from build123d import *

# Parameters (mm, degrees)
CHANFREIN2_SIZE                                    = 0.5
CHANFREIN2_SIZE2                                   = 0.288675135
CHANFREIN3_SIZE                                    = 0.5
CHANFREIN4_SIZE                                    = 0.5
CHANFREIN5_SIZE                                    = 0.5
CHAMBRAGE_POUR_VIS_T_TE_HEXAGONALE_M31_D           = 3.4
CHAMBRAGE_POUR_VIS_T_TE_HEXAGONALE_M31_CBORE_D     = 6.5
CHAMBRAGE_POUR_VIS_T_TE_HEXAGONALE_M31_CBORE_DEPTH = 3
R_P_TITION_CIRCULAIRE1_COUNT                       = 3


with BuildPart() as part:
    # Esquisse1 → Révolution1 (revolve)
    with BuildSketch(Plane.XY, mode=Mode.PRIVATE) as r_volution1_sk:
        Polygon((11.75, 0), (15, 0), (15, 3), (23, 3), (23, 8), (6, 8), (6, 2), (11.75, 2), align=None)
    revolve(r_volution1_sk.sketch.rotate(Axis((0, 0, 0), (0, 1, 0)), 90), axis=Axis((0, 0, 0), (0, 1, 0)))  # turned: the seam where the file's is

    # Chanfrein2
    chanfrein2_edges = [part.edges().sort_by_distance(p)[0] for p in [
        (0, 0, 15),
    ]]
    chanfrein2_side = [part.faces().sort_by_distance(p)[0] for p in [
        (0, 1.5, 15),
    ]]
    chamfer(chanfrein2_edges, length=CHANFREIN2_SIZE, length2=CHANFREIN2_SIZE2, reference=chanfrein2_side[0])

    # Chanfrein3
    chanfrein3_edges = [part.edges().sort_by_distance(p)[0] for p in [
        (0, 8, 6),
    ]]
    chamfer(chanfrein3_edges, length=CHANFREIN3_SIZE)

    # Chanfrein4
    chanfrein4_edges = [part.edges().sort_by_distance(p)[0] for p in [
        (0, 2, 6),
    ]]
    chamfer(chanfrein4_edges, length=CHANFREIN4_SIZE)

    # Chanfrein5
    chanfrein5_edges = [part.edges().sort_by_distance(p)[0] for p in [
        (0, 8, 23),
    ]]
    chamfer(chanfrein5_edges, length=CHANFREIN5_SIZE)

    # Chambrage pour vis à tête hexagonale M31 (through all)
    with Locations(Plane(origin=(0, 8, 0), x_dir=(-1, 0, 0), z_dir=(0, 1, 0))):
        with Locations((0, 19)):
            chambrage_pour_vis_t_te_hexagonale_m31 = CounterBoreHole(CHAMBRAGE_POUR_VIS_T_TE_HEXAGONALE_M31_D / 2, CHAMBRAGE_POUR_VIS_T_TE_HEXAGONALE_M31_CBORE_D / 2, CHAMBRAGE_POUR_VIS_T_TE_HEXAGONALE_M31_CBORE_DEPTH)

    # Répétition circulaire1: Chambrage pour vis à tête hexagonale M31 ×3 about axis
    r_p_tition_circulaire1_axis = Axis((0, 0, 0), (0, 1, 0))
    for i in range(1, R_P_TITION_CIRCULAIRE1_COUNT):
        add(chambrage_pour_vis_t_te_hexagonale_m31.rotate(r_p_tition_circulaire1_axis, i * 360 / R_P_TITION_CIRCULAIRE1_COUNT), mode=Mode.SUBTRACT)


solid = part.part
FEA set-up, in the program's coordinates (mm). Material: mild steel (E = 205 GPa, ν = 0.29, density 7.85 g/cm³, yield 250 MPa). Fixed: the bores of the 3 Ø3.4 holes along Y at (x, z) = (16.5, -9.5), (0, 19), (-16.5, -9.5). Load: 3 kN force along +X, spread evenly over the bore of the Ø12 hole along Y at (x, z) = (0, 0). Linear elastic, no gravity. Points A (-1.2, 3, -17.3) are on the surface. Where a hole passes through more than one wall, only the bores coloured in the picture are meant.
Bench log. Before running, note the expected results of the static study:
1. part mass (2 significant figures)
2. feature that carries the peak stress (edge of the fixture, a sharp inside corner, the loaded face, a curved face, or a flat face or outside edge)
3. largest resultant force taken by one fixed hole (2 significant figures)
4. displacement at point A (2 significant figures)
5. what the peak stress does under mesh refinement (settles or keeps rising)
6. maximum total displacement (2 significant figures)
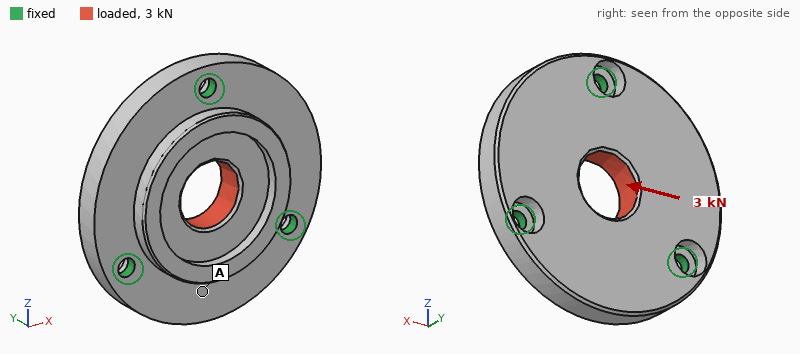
67 g
edge of the fixture
1.0 kN
1.1 µm
keeps rising
2.7 µm
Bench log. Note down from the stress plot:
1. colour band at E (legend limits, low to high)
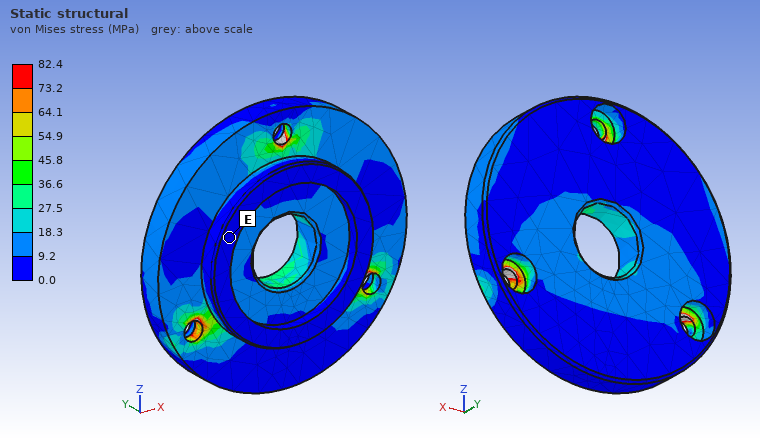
0.0 to 9.2 MPa
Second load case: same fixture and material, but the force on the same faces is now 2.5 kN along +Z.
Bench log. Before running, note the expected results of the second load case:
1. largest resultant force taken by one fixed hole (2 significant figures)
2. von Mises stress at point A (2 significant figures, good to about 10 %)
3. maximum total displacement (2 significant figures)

870 N
8.6 MPa
2.6 µm
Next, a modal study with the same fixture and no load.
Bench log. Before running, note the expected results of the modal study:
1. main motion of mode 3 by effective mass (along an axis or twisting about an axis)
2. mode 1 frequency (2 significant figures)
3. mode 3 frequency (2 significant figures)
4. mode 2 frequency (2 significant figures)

along Y
11 kHz
14 kHz
11 kHz
